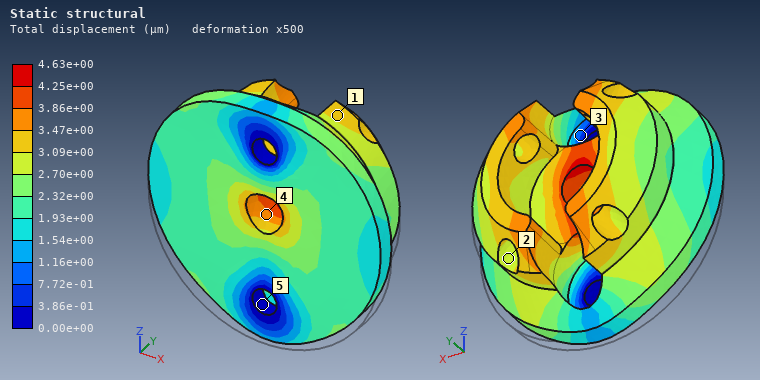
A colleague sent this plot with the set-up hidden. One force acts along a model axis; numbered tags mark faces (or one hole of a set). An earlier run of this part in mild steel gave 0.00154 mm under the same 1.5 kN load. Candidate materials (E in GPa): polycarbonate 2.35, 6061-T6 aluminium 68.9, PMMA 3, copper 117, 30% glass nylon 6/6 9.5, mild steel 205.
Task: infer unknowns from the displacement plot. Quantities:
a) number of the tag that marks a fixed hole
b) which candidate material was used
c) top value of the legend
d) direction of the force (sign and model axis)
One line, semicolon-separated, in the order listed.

5; 6061-T6 aluminium; 4.63e+00 µm; +Z
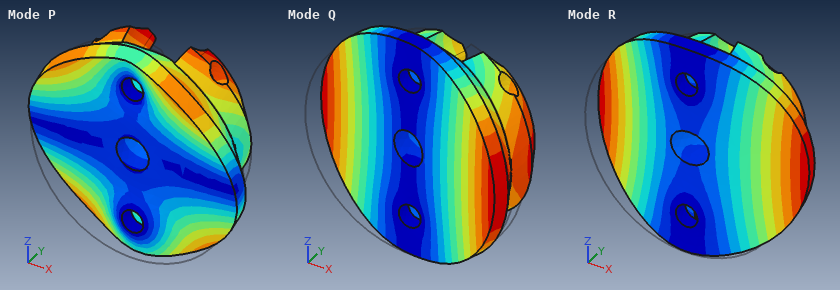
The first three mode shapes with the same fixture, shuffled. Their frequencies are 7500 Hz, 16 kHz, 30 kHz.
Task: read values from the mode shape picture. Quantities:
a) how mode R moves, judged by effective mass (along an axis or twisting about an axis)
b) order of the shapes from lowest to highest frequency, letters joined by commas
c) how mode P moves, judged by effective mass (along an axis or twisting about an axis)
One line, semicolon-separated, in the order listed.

along Y; Q, R, P; along Z
